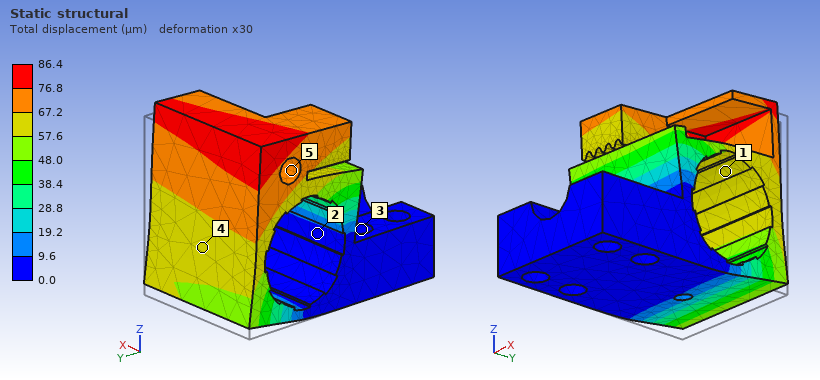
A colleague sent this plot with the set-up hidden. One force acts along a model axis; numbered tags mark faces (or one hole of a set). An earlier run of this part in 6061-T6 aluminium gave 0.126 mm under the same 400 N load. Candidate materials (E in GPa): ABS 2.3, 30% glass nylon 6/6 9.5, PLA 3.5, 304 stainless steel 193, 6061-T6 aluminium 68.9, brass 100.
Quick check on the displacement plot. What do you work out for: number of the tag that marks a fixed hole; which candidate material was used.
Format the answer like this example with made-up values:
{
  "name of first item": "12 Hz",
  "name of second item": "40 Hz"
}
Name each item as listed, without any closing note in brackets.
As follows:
{
  "number of the tag that marks a fixed hole": "3",
  "which candidate material was used": "brass"
}
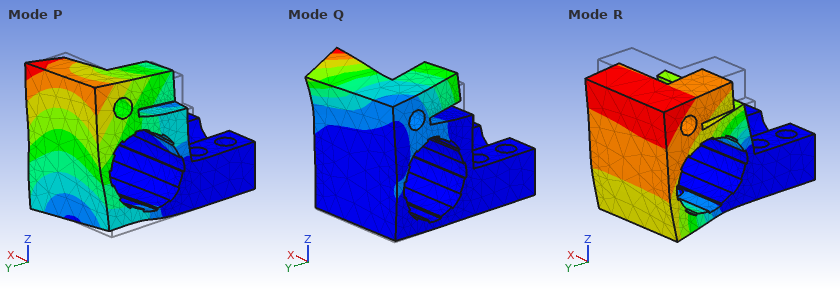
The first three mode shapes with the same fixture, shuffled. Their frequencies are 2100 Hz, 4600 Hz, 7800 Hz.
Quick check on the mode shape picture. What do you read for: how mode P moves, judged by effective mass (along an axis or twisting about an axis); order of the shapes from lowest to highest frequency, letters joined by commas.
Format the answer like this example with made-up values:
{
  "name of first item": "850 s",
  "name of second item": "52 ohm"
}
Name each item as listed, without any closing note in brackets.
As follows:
{
  "how mode P moves, judged by effective mass": "along X",
  "order of the shapes from lowest to highest frequency, letters joined by commas": "R, P, Q"
}
